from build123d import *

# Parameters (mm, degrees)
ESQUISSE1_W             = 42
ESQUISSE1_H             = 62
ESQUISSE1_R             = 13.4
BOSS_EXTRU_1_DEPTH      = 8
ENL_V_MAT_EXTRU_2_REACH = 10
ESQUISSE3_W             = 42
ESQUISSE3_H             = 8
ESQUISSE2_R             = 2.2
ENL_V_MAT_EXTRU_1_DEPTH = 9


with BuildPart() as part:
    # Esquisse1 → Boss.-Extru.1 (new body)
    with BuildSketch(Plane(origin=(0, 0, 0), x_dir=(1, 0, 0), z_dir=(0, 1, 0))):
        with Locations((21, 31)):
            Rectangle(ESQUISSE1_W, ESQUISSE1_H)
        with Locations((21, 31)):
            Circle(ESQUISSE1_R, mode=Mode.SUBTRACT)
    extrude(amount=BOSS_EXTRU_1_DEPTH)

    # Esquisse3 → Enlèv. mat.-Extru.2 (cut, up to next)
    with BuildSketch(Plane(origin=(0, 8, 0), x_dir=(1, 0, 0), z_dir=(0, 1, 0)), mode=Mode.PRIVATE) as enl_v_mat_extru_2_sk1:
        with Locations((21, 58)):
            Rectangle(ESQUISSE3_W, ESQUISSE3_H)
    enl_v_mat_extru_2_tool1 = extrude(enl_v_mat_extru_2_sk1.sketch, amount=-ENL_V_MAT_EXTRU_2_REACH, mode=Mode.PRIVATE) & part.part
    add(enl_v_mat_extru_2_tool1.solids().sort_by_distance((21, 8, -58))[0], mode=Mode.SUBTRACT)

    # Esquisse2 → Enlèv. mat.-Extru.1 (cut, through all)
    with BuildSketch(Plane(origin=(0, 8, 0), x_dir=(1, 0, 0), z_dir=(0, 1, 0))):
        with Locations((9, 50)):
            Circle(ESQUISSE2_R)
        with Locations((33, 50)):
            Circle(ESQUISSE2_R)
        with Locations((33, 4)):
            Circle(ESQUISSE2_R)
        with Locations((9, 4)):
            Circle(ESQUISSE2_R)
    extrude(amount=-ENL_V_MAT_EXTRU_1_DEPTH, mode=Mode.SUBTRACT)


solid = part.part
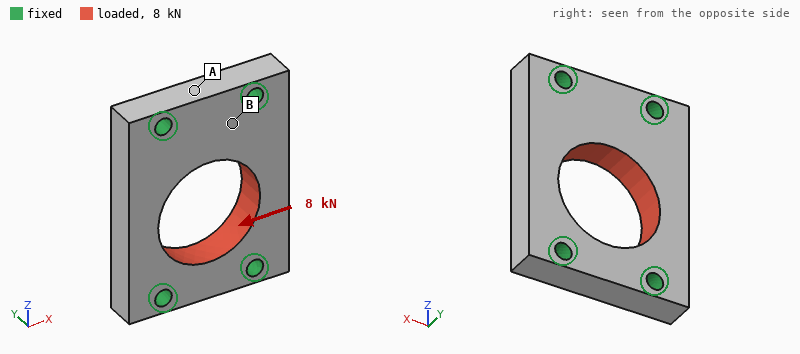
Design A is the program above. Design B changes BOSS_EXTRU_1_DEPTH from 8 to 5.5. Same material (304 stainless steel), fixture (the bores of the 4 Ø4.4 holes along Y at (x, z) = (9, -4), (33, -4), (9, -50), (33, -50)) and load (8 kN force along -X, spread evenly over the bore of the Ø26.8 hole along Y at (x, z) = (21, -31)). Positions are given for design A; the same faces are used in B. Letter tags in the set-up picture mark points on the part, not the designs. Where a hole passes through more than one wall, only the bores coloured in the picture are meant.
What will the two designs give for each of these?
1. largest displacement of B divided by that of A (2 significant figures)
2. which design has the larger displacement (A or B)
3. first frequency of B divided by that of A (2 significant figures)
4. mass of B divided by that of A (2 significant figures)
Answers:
1.5
B
0.77
0.69
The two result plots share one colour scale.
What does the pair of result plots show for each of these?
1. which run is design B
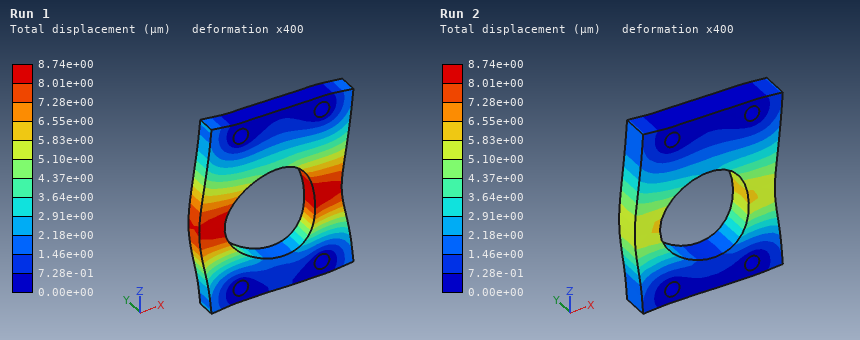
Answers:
Run 1
